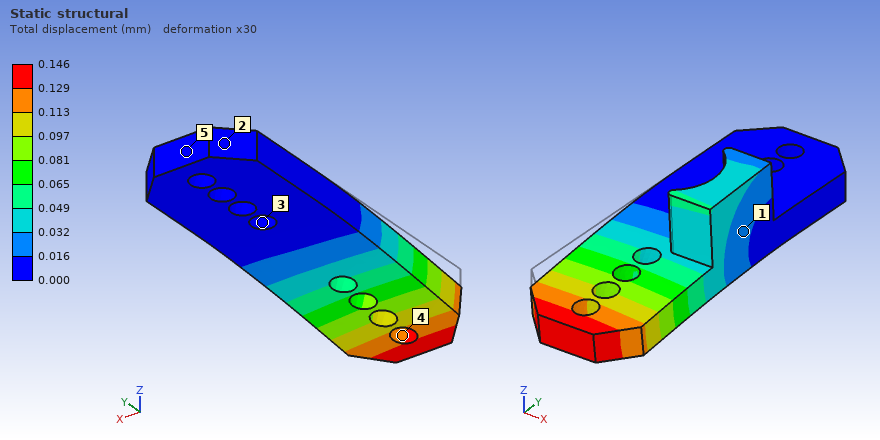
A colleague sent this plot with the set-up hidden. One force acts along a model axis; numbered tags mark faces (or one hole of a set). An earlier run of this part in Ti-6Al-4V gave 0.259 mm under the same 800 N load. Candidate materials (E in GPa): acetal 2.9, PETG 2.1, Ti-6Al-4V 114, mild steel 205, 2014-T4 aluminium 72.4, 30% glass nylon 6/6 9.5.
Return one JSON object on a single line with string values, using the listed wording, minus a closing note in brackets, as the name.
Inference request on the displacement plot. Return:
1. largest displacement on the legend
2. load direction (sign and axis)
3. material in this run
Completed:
{"largest displacement on the legend": "0.146 mm", "load direction": "-Z", "material in this run": "mild steel"}
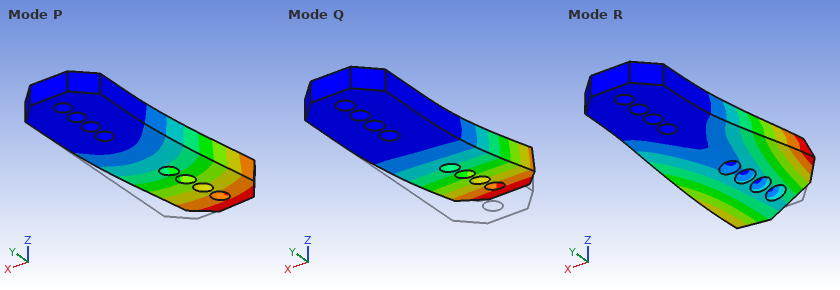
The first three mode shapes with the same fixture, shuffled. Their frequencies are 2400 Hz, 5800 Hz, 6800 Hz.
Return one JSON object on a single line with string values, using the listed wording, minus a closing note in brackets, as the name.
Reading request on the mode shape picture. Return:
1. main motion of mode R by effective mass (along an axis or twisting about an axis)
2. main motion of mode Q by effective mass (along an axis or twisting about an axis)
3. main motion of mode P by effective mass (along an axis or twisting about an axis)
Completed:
{"main motion of mode R by effective mass": "twisting about Y", "main motion of mode Q by effective mass": "along Z", "main motion of mode P by effective mass": "along X"}
